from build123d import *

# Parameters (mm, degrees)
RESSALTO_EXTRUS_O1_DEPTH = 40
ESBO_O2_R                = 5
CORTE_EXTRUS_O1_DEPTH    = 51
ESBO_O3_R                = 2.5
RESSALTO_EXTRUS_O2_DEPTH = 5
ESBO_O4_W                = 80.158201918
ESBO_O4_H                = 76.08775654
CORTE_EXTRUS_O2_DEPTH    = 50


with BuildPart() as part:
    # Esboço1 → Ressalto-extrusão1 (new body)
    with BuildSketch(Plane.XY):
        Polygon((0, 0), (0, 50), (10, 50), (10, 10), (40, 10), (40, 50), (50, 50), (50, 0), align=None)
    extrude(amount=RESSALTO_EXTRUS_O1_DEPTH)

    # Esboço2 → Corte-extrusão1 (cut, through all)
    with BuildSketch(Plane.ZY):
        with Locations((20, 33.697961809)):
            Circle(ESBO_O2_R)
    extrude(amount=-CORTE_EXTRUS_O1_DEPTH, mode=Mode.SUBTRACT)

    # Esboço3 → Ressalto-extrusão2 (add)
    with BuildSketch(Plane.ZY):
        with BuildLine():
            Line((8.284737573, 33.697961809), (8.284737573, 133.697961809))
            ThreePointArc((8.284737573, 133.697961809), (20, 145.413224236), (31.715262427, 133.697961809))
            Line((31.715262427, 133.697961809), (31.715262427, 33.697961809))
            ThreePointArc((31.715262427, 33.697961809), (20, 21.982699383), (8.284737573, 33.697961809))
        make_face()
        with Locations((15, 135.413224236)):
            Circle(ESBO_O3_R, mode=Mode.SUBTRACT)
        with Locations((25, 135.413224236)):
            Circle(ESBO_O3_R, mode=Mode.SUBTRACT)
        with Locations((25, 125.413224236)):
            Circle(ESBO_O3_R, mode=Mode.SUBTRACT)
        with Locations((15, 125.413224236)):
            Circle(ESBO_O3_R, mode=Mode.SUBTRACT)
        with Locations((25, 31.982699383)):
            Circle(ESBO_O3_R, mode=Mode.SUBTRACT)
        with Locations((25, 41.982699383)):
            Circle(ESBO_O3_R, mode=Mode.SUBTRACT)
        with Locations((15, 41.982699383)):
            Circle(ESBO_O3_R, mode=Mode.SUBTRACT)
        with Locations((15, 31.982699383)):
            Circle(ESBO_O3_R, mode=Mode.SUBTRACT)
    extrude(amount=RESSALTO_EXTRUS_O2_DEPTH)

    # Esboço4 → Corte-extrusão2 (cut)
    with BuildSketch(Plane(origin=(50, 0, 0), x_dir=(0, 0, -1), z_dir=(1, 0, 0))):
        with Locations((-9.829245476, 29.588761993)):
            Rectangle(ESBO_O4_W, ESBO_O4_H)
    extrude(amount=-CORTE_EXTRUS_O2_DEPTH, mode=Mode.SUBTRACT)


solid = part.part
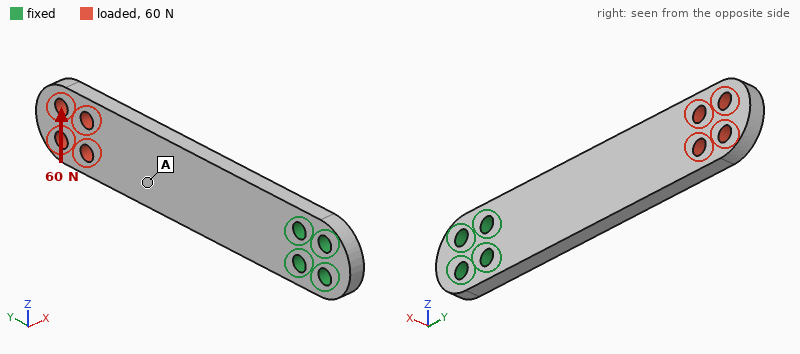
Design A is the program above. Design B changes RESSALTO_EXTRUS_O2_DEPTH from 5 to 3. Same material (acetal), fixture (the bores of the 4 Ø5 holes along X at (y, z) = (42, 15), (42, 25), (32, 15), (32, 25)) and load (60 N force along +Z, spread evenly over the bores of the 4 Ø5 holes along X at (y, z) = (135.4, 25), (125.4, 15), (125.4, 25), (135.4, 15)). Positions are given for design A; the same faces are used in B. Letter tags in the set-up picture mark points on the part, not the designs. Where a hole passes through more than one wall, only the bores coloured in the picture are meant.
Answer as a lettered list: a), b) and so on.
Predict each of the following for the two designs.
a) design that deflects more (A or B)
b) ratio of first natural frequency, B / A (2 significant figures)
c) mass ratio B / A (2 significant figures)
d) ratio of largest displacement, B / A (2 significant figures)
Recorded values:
a) B
b) 0.61
c) 0.60
d) 1.7
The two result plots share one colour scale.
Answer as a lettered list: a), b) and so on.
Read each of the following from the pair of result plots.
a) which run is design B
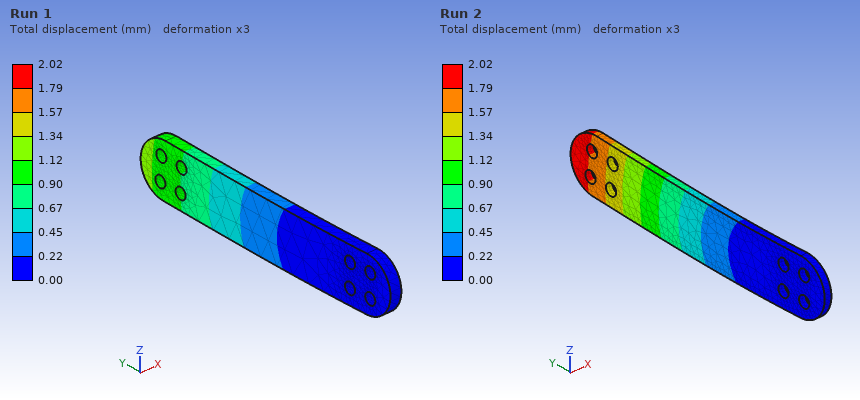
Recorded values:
a) Run 2
